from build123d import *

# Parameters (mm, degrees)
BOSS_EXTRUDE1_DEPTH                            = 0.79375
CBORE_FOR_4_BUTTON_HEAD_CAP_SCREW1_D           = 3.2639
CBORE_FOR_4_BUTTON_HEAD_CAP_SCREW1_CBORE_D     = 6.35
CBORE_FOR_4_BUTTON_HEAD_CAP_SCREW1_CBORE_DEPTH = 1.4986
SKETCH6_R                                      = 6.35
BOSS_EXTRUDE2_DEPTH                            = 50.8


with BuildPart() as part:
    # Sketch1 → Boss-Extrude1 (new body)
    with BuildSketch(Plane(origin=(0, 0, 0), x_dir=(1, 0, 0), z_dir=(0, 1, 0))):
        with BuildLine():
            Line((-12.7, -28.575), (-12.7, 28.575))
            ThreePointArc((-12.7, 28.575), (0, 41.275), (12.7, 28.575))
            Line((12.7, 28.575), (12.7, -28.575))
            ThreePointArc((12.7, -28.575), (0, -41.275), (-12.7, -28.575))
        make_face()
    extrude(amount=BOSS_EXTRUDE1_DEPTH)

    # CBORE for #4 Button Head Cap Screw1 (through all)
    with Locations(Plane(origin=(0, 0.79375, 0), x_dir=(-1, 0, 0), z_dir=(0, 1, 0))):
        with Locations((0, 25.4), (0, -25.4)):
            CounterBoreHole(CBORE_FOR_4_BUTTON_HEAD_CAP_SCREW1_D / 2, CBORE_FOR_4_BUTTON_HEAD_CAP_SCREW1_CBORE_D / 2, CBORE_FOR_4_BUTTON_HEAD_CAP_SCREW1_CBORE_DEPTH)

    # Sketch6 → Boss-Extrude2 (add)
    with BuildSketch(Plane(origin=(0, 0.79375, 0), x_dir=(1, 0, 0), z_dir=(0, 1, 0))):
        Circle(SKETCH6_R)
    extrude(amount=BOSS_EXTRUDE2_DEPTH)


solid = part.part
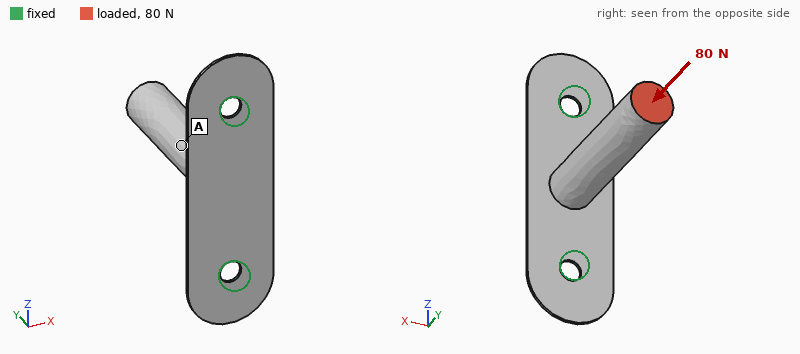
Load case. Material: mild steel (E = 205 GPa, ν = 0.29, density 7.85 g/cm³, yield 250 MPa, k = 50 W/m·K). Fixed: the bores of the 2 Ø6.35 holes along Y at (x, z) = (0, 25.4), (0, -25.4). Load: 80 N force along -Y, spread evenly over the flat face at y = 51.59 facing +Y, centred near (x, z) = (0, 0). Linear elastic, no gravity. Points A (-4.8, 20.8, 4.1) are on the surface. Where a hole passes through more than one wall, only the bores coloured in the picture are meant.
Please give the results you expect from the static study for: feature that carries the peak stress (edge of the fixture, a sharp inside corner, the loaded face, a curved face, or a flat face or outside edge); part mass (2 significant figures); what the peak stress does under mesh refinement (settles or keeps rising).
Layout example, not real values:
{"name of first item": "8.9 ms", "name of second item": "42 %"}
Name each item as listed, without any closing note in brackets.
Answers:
{"feature that carries the peak stress": "edge of the fixture", "part mass": "62 g", "what the peak stress does under mesh refinement": "keeps rising"}
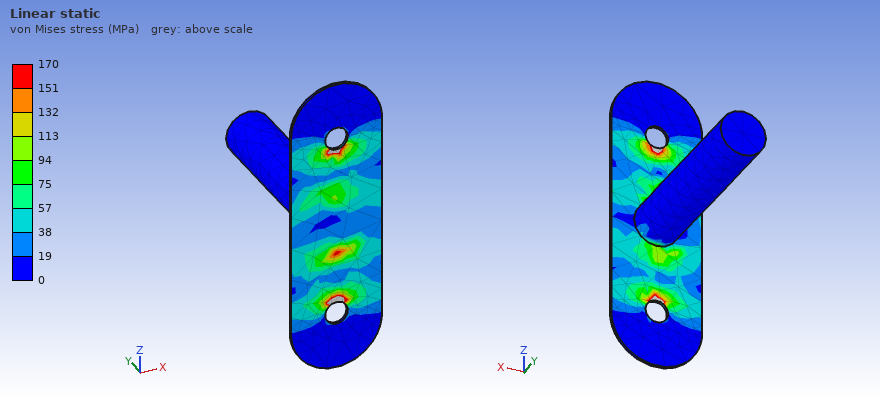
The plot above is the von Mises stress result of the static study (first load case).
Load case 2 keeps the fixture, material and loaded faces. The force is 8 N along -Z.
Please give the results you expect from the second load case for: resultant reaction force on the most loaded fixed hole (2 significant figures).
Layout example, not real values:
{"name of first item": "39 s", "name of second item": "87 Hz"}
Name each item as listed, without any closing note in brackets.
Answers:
{"resultant reaction force on the most loaded fixed hole": "13 N"}
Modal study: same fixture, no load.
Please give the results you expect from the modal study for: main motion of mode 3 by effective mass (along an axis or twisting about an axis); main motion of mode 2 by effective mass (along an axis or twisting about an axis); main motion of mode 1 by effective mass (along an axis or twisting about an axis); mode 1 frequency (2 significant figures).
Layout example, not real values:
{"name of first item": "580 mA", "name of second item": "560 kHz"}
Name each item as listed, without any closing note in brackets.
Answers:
{"main motion of mode 3 by effective mass": "along Y", "main motion of mode 2 by effective mass": "along Z", "main motion of mode 1 by effective mass": "along X", "mode 1 frequency": "170 Hz"}
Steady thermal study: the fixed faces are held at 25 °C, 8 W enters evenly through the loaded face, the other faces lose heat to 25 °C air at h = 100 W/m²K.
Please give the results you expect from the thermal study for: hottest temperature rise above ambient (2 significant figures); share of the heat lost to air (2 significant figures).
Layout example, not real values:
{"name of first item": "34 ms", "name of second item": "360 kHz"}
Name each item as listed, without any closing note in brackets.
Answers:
{"hottest temperature rise above ambient": "50 K", "share of the heat lost to air": "91 %"}
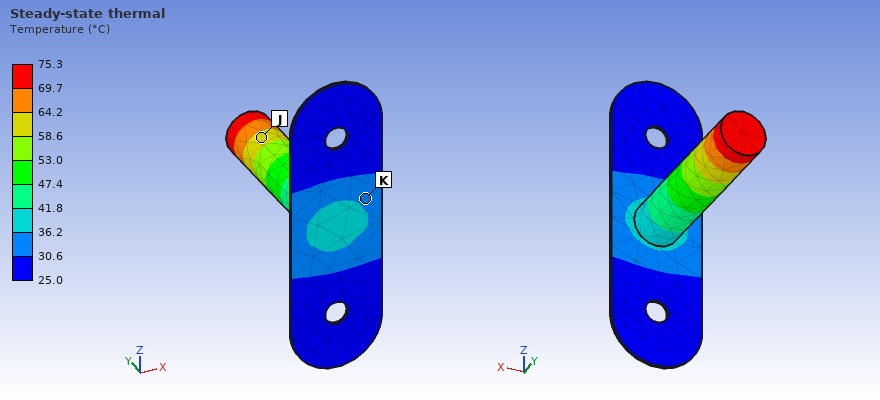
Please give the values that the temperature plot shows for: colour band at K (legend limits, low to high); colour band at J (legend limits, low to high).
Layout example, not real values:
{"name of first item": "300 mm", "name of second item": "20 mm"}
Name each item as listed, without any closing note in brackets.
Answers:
{"colour band at K": "30.6 to 36.2 °C", "colour band at J": "58.6 to 64.2 °C"}
